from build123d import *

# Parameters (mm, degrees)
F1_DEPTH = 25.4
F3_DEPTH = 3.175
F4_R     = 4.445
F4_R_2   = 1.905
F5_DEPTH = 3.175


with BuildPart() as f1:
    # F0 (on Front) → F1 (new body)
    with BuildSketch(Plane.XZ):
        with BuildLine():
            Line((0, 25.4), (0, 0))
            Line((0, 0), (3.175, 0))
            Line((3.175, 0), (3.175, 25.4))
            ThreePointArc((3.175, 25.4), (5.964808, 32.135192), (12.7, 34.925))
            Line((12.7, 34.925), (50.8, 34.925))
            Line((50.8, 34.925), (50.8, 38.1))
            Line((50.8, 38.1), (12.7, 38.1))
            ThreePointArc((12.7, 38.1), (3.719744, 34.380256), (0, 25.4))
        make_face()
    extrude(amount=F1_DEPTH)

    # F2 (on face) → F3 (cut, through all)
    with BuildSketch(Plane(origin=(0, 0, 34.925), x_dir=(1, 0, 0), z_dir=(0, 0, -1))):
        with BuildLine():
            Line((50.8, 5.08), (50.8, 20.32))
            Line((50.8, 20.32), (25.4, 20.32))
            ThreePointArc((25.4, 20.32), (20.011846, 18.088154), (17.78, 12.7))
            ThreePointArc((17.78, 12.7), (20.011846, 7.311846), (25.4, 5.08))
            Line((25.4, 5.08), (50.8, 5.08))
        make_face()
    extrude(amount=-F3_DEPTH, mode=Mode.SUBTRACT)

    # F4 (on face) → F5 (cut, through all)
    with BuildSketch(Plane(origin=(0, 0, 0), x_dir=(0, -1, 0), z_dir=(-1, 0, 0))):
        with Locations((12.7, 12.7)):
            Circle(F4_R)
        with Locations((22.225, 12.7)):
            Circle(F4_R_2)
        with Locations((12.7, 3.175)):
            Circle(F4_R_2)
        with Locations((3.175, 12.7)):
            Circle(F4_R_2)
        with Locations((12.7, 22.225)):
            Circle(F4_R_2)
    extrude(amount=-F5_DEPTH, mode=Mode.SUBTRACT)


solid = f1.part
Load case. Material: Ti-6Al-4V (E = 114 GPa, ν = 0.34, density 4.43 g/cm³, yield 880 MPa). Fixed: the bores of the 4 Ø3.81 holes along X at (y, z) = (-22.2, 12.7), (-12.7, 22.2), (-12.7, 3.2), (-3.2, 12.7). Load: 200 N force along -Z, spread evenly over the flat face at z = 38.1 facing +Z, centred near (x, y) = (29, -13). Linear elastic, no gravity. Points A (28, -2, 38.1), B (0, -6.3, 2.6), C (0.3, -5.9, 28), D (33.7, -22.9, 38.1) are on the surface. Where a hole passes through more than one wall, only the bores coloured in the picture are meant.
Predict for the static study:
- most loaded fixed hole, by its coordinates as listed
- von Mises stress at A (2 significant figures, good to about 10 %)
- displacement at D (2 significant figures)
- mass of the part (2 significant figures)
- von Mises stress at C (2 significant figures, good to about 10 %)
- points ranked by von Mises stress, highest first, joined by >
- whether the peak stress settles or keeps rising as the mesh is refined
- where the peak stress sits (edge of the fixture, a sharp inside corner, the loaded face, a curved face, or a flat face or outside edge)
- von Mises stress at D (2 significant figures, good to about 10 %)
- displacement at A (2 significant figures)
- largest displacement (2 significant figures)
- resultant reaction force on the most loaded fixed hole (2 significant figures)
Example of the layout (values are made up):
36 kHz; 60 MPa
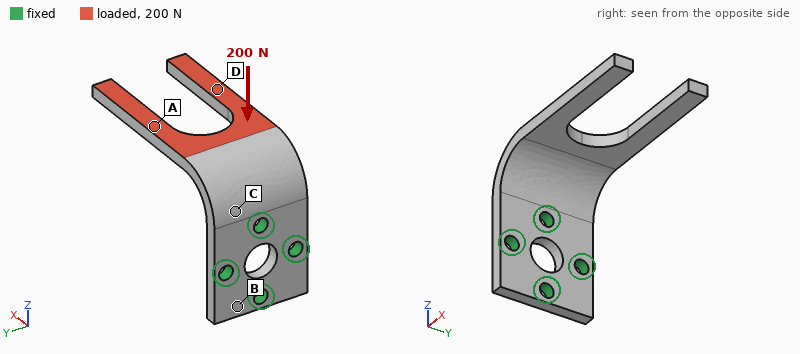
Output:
(-12.7, 22.2); 63 MPa; 0.46 mm; 21 g; 94 MPa; C > A > D > B; keeps rising; edge of the fixture; 36 MPa; 0.35 mm; 0.81 mm; 310 N
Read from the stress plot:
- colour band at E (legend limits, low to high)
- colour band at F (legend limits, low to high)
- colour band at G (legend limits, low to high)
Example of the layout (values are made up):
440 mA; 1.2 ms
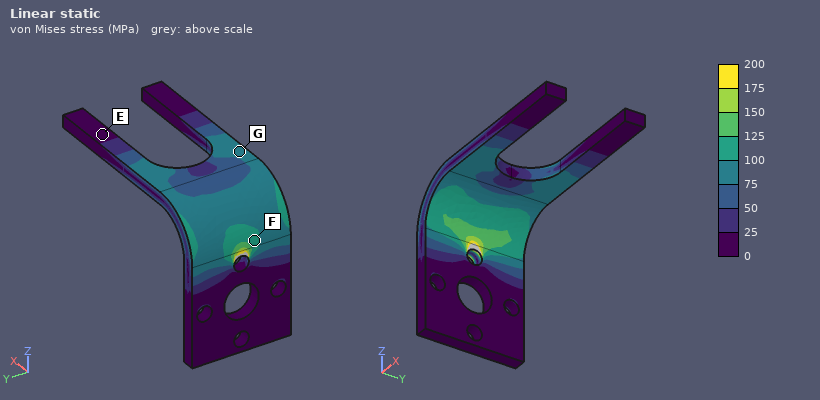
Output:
0 to 25 MPa; 100 to 125 MPa; 75 to 100 MPa
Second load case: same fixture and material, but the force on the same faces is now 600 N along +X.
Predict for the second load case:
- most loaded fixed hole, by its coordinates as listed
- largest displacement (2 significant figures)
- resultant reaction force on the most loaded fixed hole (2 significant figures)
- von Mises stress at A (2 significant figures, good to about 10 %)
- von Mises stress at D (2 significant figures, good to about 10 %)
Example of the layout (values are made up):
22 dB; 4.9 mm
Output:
(-12.7, 22.2); 0.62 mm; 960 N; 35 MPa; 26 MPa
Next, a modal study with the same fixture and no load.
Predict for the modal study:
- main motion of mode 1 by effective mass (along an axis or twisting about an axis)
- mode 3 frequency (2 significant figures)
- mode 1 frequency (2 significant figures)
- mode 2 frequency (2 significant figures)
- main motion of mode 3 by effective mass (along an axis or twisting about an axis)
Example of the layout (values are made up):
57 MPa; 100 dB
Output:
along Z; 2000 Hz; 1200 Hz; 1700 Hz; along Y
